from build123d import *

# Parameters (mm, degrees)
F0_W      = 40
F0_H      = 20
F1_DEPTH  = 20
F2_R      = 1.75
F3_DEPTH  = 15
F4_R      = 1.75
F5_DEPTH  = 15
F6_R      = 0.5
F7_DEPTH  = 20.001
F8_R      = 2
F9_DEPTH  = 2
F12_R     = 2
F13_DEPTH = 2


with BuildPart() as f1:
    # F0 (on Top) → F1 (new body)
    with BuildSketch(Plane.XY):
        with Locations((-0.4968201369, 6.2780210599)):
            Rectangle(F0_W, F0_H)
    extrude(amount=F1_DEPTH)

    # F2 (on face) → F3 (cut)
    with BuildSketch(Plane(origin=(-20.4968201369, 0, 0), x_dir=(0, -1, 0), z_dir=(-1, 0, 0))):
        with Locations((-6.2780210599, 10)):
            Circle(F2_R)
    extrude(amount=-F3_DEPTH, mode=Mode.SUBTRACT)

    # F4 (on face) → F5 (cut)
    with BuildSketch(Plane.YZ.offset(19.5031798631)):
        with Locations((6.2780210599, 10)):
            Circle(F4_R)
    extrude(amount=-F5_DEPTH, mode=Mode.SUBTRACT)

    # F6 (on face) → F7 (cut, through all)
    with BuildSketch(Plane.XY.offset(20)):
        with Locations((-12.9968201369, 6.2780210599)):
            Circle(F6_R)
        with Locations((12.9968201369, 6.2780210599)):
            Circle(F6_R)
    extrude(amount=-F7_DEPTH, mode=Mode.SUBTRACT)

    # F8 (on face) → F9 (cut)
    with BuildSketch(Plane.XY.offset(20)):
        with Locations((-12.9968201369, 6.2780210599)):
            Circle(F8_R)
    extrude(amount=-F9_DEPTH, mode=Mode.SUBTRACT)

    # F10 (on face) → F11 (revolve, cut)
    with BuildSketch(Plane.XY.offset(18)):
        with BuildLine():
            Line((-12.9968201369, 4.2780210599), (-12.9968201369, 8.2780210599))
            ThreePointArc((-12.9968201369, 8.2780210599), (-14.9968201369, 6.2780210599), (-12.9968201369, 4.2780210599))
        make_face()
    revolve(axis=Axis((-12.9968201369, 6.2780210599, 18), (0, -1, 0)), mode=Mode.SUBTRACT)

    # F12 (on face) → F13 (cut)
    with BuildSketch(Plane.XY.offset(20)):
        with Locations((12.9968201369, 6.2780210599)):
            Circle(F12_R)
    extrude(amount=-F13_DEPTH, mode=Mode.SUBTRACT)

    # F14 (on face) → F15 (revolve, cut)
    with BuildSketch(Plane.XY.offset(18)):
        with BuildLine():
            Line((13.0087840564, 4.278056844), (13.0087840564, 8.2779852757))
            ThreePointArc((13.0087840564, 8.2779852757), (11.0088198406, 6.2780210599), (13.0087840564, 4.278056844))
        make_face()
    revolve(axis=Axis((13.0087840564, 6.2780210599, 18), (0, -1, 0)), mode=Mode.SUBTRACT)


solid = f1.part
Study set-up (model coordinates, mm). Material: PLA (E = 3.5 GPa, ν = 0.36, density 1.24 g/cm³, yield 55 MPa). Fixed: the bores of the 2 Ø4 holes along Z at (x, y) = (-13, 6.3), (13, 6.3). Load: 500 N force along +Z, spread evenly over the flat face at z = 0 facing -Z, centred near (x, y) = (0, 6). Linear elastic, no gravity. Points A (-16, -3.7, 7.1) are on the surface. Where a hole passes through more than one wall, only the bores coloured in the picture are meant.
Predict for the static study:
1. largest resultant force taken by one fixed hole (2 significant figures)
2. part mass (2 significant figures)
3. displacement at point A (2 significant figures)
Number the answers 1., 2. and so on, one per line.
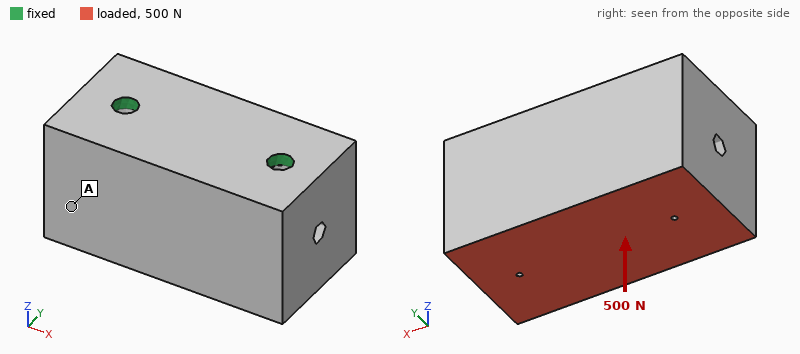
1. 260 N
2. 19 g
3. 11 µm
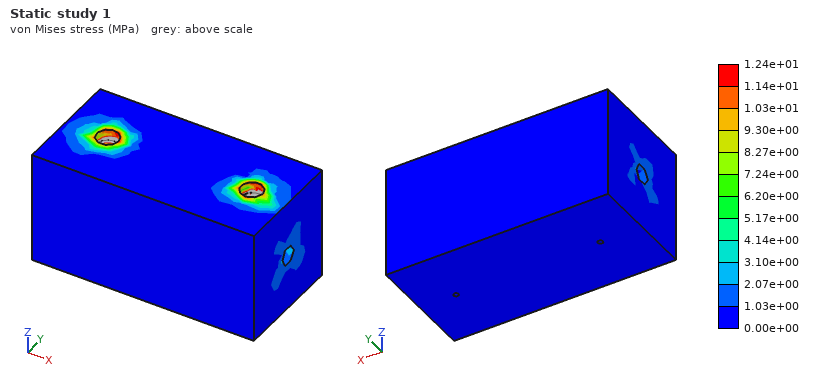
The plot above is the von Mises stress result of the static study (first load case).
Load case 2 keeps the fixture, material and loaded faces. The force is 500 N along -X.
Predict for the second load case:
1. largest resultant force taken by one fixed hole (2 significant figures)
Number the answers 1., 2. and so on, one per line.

1. 430 N
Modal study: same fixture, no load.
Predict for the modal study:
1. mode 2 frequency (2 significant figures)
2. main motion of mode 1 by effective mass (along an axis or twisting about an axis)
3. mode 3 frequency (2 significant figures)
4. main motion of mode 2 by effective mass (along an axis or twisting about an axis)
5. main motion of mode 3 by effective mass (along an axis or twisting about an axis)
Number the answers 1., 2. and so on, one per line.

1. 5500 Hz
2. along Y
3. 6200 Hz
4. along X
5. twisting about Z
